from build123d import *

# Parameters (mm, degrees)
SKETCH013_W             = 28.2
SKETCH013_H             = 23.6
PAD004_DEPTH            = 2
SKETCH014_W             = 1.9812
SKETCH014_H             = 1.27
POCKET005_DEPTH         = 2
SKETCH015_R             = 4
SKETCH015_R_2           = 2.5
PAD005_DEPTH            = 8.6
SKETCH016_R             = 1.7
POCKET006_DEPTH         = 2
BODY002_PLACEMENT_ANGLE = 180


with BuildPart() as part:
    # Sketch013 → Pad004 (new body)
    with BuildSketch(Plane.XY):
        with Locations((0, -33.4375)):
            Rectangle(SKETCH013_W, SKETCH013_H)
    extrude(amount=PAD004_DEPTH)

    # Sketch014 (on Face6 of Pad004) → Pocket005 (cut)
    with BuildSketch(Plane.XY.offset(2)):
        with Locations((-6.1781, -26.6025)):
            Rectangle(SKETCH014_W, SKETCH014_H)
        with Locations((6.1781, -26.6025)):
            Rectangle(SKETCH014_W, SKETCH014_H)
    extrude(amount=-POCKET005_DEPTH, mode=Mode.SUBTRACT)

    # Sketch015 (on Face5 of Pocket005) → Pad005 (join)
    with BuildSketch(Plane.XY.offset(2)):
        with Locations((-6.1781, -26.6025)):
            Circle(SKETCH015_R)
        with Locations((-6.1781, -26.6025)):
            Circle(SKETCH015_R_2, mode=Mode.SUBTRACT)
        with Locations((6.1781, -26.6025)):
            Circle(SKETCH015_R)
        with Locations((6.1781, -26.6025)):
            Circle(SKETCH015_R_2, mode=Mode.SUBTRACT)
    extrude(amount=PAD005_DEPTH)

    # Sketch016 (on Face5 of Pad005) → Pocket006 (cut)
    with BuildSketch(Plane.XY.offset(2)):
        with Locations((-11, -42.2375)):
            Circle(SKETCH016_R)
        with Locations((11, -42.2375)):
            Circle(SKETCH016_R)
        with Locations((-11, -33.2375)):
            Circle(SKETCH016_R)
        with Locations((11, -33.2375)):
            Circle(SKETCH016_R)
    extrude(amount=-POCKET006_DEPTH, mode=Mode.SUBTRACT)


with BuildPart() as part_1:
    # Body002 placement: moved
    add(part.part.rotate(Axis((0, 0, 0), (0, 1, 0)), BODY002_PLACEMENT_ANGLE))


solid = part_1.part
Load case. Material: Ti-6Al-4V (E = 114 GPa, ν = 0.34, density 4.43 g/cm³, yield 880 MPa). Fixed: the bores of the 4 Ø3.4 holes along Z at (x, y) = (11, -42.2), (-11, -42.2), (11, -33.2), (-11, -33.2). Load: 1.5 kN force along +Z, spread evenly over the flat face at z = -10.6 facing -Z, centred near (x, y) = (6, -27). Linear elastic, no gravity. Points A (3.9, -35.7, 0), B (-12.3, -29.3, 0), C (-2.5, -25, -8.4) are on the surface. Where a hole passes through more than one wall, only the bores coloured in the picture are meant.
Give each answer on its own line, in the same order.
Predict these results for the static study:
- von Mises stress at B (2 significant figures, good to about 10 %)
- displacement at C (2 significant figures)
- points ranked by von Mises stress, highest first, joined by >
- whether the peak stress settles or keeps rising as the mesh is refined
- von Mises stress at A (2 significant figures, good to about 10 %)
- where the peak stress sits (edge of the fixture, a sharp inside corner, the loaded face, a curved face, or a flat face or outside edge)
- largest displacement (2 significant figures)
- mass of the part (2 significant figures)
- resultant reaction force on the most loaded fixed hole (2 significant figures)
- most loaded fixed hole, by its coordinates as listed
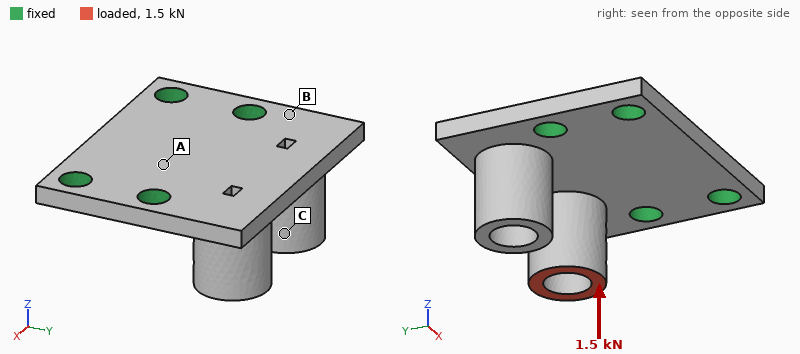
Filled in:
260 MPa
0.16 mm
B > A > C
keeps rising
160 MPa
edge of the fixture
0.26 mm
7.9 g
1.4 kN
(11, -33.2)
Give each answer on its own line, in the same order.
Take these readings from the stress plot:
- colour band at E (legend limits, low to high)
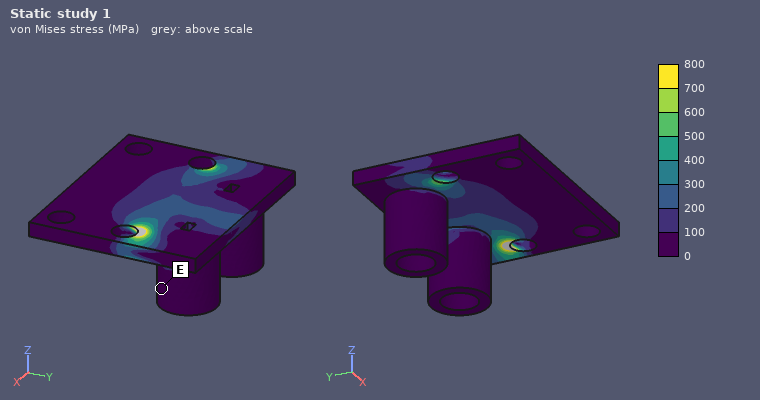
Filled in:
0 to 100 MPa
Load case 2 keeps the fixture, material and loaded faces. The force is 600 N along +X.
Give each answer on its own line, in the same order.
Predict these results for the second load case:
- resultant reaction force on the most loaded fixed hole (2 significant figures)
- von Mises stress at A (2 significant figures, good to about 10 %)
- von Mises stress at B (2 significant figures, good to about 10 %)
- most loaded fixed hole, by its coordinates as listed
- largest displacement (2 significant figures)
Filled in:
460 N
74 MPa
100 MPa
(11, -33.2)
0.10 mm
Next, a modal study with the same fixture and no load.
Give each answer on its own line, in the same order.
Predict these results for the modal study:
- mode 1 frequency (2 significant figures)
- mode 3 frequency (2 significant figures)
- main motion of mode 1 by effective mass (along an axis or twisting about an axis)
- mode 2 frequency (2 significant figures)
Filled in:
7100 Hz
15 kHz
along Z
13 kHz
